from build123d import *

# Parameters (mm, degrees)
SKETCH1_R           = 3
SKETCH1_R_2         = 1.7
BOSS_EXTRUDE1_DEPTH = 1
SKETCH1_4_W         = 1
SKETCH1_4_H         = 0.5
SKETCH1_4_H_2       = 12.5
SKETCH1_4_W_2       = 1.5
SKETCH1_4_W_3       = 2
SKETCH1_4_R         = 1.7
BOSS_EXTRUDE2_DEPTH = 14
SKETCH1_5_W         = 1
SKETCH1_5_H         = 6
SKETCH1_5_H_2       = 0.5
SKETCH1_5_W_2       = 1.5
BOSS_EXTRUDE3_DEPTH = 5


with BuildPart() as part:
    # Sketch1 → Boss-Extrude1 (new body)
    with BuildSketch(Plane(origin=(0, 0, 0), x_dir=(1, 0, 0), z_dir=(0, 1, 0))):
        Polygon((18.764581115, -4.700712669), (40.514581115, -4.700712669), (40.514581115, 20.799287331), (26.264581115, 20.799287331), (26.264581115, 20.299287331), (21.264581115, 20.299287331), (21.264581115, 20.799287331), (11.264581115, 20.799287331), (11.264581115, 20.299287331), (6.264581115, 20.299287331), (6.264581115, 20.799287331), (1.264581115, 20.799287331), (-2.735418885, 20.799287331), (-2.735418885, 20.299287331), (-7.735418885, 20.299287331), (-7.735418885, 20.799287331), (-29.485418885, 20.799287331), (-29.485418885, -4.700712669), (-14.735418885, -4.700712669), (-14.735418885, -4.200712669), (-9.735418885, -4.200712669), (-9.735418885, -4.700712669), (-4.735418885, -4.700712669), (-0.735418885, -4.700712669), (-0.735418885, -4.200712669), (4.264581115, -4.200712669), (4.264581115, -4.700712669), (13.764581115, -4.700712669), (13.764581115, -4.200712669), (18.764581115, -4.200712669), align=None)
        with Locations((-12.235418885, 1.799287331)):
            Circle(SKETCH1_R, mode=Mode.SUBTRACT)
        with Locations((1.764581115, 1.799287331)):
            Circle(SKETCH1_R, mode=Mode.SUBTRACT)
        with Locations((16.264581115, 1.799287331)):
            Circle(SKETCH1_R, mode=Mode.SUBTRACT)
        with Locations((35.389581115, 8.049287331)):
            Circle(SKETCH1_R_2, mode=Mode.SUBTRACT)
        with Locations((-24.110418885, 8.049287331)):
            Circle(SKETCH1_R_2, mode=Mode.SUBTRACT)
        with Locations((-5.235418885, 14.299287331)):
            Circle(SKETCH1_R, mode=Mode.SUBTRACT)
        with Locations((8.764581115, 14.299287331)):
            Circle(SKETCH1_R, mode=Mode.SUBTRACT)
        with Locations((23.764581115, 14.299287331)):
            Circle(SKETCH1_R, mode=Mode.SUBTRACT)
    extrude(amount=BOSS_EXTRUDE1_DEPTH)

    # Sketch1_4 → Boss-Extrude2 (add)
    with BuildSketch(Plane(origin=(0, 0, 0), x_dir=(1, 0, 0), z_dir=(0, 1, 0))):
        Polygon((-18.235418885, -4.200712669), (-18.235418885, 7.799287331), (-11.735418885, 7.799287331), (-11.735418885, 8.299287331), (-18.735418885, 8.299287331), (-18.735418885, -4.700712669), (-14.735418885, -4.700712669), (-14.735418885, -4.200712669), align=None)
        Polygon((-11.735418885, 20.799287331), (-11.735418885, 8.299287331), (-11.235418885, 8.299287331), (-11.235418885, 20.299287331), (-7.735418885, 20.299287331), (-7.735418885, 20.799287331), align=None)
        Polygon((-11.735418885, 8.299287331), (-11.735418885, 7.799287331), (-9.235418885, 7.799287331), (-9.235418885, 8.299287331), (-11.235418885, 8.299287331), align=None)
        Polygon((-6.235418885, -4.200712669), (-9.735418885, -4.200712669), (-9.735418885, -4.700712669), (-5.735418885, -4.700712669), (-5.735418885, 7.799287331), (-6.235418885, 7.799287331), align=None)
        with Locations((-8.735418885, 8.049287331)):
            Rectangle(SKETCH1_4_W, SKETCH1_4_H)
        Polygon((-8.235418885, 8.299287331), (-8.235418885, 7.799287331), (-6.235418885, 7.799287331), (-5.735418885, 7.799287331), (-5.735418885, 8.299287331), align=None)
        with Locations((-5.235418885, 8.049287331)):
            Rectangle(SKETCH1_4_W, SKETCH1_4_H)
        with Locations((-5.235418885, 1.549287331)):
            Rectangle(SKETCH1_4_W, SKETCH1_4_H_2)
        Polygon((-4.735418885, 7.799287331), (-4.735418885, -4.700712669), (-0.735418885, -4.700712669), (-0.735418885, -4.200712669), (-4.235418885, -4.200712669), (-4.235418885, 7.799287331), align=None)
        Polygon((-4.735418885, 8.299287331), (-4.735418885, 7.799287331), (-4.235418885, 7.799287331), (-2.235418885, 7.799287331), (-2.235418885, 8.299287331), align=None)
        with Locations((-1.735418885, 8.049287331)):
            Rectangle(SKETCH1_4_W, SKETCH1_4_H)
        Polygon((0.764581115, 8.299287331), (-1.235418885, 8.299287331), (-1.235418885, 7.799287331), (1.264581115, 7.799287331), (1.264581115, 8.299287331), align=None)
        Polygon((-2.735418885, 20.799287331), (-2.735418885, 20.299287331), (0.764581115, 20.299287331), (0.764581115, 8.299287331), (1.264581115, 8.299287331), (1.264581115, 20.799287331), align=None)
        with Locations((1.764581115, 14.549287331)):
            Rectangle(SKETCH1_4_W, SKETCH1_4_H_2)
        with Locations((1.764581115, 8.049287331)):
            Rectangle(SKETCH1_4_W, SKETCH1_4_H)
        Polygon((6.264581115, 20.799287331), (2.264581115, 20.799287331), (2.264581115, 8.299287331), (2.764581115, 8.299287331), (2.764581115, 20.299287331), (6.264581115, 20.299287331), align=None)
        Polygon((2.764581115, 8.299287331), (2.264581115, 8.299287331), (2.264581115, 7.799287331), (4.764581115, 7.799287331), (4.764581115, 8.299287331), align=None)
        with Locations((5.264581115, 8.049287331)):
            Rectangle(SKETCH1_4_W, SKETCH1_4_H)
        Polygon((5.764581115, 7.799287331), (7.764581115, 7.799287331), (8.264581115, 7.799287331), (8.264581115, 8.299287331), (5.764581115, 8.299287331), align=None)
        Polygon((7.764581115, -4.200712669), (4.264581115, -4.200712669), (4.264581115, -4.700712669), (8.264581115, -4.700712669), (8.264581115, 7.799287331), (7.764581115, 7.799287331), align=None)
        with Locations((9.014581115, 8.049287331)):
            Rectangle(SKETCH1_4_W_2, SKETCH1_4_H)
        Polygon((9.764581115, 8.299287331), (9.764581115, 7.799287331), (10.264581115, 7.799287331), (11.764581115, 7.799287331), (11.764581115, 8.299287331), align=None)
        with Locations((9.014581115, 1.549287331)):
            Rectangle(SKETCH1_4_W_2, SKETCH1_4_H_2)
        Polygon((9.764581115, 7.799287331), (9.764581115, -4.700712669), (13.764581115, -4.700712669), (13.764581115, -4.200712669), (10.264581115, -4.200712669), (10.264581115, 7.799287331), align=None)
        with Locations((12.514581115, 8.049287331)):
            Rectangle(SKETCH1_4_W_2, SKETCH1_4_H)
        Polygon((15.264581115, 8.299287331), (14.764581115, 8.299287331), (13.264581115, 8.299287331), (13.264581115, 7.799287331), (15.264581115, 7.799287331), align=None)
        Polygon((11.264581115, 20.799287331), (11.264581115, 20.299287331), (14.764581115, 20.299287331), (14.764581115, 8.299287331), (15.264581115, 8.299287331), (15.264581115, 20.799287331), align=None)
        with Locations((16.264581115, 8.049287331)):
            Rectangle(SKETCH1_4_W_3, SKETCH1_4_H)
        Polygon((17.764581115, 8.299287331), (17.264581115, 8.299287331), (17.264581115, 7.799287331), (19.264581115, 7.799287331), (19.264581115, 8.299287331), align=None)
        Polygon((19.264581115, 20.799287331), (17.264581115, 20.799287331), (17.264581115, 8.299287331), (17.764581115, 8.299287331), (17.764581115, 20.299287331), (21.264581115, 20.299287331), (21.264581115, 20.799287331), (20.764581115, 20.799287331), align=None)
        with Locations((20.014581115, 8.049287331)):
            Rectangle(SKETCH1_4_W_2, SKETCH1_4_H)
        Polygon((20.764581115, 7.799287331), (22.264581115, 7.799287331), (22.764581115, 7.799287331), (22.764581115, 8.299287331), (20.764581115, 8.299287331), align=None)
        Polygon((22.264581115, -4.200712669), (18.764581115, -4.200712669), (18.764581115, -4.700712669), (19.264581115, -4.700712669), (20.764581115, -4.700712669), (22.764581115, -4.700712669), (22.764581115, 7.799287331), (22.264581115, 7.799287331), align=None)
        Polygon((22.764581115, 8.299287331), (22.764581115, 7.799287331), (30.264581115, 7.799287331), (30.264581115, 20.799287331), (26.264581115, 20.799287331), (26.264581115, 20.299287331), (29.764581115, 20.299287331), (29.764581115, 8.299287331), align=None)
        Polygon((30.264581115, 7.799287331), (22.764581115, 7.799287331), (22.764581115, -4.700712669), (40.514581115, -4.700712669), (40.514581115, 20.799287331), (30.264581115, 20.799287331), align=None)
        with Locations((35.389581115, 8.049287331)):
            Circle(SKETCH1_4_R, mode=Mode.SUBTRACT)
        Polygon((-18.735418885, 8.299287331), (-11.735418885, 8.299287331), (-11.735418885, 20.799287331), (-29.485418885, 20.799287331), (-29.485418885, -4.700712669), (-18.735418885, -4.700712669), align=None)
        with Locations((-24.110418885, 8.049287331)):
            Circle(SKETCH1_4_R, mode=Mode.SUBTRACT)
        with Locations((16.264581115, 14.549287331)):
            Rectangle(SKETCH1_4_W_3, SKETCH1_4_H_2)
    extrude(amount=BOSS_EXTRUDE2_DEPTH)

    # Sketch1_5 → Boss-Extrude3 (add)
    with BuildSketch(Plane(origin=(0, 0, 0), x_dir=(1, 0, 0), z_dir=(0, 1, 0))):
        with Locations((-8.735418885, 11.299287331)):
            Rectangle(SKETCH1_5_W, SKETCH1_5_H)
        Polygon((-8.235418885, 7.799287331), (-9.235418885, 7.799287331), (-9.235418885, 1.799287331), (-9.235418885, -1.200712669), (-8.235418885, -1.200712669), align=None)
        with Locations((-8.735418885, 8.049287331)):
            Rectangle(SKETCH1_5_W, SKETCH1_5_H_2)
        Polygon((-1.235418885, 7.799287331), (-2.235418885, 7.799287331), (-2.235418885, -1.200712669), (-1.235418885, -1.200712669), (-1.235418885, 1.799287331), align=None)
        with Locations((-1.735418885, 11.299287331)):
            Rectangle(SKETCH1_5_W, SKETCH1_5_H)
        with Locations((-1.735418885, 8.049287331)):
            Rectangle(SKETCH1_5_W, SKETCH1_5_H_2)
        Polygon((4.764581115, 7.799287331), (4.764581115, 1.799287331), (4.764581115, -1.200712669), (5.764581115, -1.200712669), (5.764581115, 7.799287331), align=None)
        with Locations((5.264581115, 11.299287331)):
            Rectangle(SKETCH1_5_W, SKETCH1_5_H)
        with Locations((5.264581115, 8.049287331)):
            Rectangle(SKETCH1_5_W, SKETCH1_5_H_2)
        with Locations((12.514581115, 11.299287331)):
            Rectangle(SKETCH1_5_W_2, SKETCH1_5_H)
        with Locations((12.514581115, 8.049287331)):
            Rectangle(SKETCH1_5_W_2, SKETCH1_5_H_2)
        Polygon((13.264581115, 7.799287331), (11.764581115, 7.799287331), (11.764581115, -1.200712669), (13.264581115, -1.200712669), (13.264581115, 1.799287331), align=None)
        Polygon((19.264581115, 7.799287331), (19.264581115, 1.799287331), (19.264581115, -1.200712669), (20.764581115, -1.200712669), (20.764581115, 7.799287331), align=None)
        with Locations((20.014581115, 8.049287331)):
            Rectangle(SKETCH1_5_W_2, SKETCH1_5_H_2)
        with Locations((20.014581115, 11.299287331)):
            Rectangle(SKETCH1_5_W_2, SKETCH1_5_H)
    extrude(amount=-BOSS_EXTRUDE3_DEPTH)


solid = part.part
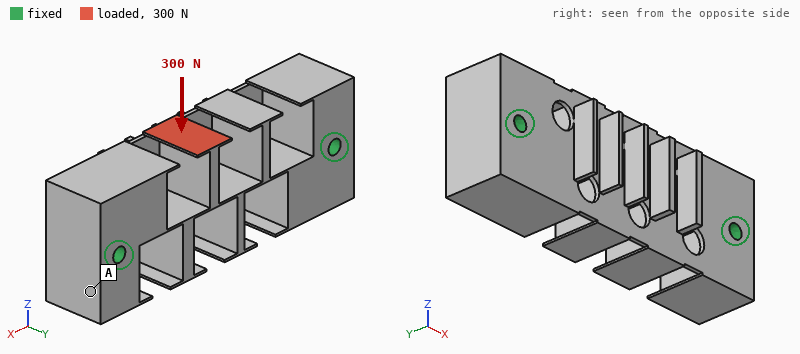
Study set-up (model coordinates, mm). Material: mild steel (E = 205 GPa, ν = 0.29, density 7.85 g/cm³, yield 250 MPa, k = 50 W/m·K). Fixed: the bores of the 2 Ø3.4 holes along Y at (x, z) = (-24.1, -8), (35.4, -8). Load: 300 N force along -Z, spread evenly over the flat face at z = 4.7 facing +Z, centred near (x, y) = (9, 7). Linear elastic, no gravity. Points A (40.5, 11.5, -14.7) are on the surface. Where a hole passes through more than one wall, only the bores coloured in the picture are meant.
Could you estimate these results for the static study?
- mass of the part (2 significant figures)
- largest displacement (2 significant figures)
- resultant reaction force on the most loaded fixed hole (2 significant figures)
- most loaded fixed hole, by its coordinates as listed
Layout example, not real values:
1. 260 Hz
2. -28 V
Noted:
1. 110 g
2. 57 µm
3. 180 N
4. (35.4, -8)
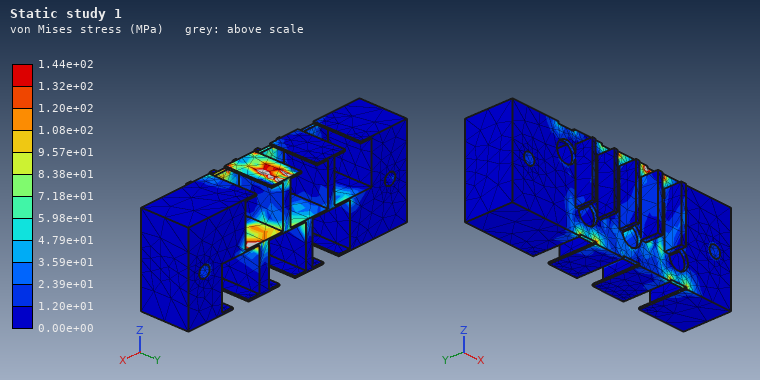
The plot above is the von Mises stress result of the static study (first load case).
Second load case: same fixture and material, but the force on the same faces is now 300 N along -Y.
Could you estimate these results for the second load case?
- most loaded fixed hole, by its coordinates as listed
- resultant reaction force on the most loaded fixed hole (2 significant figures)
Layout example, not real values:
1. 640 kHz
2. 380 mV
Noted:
1. (35.4, -8)
2. 190 N
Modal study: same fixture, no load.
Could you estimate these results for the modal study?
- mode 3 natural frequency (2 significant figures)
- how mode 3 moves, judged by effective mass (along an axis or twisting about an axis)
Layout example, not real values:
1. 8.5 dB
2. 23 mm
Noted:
1. 8100 Hz
2. along Y
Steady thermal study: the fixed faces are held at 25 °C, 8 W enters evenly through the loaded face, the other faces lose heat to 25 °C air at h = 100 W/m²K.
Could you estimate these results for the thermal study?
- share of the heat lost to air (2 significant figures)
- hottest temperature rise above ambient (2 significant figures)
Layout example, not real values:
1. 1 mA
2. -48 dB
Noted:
1. 78 %
2. 69 K
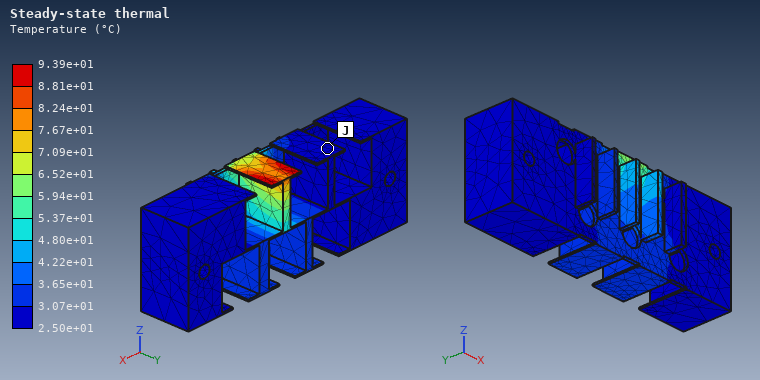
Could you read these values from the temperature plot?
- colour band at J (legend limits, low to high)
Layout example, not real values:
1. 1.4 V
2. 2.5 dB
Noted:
1. 2.50e+01 to 3.07e+01 °C
